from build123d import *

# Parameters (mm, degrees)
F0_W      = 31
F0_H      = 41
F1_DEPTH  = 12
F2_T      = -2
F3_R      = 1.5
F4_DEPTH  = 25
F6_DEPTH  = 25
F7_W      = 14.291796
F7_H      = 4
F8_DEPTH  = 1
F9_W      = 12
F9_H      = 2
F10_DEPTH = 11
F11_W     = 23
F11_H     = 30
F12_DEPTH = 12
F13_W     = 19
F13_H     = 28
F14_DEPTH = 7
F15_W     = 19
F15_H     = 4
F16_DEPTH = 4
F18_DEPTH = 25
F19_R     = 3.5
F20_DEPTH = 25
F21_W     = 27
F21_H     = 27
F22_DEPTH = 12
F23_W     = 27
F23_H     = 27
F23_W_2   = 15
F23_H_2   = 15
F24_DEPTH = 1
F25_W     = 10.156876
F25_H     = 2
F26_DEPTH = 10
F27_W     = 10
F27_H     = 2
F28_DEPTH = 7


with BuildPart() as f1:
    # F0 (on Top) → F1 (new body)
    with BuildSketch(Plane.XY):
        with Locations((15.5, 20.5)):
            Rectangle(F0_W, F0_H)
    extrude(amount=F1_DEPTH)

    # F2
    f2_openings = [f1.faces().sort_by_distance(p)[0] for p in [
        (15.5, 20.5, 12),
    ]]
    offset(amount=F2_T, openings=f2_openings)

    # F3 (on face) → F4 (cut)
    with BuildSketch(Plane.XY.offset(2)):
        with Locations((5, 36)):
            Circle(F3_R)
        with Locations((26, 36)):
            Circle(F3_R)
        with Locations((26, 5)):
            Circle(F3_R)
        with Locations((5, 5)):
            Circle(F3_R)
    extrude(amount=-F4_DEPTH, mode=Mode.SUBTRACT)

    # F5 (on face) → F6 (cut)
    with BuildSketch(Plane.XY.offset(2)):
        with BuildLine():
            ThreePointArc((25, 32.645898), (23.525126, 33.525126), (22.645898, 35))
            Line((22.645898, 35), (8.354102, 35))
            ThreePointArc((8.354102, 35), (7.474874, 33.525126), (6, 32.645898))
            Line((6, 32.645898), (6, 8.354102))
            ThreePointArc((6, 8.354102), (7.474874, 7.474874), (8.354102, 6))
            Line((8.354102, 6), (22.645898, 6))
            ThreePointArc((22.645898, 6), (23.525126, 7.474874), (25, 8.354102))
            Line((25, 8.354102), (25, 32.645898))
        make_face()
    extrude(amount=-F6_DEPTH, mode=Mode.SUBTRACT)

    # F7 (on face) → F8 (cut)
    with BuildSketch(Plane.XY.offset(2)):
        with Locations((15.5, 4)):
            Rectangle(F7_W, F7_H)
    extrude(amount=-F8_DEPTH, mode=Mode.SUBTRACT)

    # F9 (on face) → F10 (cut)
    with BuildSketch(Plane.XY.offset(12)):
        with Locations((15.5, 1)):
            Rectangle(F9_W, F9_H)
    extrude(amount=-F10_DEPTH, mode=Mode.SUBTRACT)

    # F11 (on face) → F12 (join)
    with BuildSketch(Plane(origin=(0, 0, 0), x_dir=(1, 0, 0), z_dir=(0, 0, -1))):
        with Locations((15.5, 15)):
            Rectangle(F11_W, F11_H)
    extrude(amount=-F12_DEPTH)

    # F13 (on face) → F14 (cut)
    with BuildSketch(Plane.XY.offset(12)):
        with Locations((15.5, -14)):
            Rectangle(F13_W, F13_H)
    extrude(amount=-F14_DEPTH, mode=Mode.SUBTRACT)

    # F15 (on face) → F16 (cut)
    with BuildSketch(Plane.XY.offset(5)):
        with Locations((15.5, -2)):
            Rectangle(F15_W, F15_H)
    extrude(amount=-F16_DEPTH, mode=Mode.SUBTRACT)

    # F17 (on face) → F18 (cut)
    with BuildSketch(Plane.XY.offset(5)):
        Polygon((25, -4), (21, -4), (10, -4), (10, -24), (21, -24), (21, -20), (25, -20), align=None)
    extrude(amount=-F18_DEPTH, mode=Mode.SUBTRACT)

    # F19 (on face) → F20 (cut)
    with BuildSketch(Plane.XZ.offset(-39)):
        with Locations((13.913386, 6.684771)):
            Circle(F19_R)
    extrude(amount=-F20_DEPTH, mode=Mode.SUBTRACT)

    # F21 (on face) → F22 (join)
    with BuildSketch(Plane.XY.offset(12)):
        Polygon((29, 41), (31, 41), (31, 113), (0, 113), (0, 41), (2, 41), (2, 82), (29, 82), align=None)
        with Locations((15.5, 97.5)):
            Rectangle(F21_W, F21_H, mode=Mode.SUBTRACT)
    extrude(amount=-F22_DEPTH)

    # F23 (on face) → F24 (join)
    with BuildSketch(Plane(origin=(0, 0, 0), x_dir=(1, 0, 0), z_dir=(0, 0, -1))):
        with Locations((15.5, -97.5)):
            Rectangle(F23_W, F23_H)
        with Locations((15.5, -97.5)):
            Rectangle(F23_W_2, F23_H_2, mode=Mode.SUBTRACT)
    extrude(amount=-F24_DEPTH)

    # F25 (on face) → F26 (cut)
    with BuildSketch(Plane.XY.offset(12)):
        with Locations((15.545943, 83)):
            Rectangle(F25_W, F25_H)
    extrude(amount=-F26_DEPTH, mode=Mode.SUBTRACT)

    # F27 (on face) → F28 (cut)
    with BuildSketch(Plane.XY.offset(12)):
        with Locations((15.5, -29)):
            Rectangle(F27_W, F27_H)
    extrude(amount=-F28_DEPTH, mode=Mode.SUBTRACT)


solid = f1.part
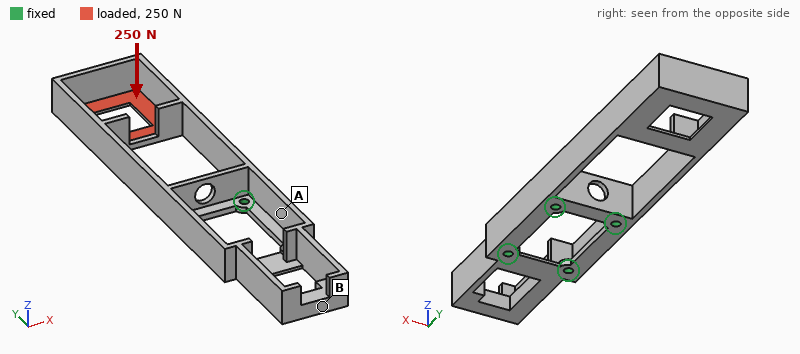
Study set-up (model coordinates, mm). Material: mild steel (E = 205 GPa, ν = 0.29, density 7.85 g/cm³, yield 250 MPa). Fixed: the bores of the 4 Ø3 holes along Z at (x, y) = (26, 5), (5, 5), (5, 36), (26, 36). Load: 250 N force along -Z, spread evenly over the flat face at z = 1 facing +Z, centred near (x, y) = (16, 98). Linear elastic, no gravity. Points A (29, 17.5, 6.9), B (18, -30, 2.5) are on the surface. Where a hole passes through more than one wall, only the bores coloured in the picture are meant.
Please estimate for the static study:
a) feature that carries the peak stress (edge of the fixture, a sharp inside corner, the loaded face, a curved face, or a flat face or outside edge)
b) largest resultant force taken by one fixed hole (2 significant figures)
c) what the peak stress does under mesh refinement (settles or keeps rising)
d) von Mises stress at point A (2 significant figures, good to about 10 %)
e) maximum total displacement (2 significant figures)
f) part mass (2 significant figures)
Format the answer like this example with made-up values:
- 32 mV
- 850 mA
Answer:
- edge of the fixture
- 520 N
- keeps rising
- 29 MPa
- 0.28 mm
- 90 g
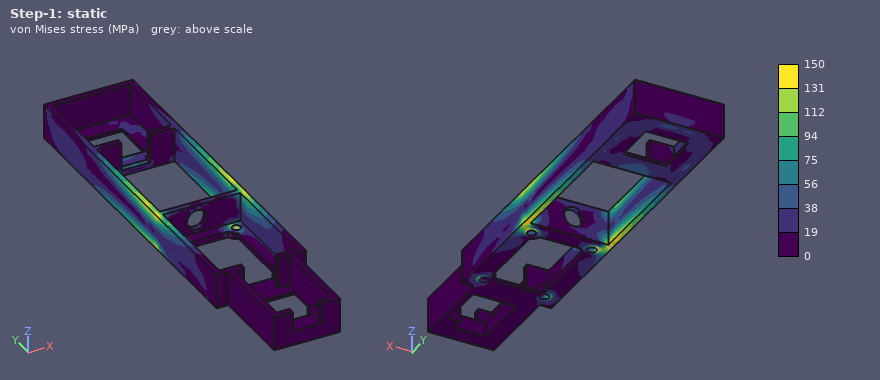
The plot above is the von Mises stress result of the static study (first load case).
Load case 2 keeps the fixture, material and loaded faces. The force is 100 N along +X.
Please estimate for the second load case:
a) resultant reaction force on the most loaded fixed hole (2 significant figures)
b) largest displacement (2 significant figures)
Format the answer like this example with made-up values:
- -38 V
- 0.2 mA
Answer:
- 110 N
- 0.25 mm
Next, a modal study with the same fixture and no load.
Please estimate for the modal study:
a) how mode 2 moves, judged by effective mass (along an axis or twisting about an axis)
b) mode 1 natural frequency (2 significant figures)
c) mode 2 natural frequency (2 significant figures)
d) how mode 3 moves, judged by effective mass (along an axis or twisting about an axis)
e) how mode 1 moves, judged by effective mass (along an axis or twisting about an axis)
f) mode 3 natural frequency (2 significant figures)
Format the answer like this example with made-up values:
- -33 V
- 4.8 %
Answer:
- along Z
- 590 Hz
- 1000 Hz
- twisting about Y
- along X
- 1600 Hz
